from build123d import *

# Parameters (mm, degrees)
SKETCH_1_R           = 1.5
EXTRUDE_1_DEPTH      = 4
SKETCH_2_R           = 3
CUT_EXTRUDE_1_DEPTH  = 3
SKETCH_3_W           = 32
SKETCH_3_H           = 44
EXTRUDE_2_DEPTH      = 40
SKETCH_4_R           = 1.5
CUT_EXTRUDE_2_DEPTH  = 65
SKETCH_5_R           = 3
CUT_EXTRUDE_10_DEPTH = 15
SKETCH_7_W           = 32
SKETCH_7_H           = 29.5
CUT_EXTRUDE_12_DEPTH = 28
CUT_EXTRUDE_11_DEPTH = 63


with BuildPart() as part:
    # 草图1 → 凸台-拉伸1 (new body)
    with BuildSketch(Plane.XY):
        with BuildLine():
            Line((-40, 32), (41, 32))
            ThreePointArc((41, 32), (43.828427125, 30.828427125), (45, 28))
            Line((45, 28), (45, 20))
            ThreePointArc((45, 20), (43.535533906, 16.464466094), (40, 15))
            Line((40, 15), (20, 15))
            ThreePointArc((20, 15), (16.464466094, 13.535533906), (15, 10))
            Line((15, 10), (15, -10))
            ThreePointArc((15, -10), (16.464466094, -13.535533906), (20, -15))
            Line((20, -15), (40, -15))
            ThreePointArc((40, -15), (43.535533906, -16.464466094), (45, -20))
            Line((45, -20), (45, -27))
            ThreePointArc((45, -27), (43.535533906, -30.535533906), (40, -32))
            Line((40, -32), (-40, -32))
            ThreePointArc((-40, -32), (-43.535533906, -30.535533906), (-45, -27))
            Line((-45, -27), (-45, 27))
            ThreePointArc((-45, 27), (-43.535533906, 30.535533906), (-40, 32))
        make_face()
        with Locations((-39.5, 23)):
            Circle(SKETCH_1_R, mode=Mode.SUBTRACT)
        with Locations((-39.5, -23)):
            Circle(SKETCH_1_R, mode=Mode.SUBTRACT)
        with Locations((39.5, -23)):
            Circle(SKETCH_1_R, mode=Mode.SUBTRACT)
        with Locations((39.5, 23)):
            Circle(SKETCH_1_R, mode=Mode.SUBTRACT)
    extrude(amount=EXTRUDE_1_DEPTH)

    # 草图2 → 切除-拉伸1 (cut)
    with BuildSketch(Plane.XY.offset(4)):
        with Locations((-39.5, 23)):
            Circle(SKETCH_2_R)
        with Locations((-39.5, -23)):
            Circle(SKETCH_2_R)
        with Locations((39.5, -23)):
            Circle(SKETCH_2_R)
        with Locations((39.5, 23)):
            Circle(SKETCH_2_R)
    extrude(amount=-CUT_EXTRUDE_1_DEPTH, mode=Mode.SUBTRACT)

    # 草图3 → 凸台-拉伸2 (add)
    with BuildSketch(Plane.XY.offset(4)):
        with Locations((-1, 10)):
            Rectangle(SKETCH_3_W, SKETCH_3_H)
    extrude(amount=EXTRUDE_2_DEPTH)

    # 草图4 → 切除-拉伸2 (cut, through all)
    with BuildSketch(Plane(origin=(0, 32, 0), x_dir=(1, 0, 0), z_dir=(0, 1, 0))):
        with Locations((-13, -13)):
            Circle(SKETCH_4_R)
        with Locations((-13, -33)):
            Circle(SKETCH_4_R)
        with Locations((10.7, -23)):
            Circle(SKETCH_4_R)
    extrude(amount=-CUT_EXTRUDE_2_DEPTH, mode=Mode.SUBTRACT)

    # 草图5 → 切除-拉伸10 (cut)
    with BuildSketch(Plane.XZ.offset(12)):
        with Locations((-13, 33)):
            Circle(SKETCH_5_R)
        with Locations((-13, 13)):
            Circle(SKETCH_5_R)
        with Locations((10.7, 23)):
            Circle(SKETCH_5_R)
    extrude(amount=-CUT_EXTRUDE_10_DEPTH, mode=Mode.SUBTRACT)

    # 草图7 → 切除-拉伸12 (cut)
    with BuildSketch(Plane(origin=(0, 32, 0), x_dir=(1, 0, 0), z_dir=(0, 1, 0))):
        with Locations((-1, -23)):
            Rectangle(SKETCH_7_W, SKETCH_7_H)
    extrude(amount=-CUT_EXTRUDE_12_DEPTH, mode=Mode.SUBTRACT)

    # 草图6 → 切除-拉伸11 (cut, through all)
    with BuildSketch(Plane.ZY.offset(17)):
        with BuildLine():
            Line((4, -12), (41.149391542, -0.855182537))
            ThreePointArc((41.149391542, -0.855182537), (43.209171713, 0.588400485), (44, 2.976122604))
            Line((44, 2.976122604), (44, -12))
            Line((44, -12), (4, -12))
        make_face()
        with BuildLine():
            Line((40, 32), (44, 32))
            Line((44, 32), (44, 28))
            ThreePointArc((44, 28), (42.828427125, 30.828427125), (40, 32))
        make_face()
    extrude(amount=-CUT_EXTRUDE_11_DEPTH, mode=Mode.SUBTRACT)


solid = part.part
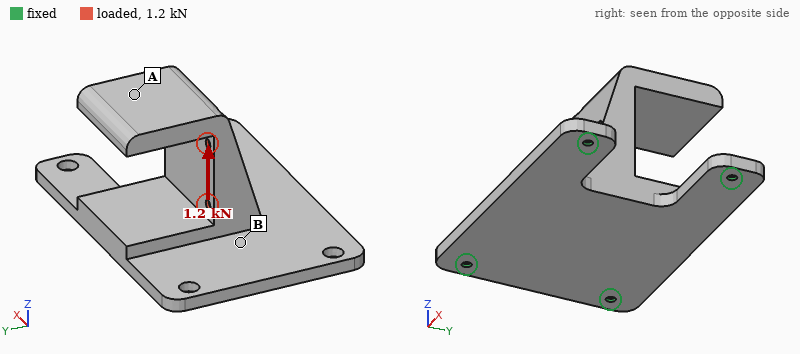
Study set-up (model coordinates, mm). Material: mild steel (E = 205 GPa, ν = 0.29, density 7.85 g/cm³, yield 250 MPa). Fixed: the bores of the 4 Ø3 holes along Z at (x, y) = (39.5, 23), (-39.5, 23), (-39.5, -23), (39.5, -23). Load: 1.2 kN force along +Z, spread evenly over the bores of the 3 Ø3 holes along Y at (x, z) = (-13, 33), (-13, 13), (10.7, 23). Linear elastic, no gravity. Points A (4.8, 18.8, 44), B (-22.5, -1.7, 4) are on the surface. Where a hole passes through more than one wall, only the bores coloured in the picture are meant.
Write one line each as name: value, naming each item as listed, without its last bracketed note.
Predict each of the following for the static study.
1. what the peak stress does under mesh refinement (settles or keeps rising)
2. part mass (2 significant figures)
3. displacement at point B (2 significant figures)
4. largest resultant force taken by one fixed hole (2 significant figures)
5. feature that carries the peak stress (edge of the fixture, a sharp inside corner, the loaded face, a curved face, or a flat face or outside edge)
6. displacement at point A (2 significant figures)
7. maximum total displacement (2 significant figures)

what the peak stress does under mesh refinement: keeps rising
part mass: 320 g
displacement at point B: 39 µm
largest resultant force taken by one fixed hole: 1.1 kN
feature that carries the peak stress: edge of the fixture
displacement at point A: 55 µm
maximum total displacement: 59 µm
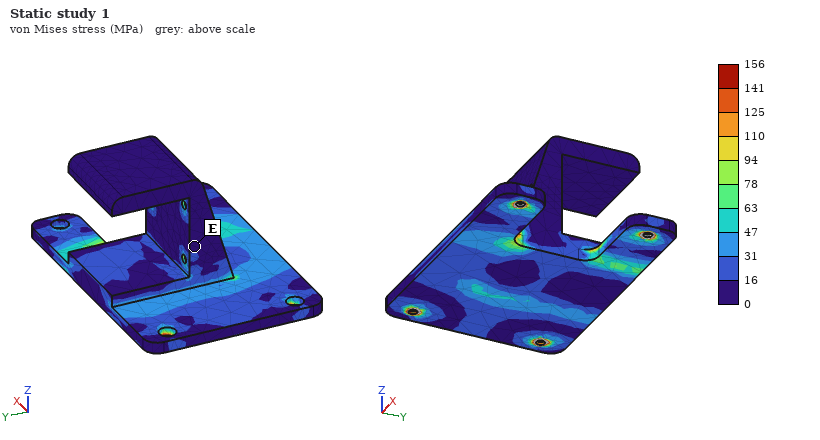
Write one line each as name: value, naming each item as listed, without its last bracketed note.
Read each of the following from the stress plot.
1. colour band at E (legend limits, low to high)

colour band at E: 0 to 16 MPa
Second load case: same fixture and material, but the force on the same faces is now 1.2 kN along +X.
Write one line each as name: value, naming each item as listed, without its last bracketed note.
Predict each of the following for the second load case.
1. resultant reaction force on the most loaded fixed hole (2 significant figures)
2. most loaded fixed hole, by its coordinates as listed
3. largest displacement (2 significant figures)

resultant reaction force on the most loaded fixed hole: 550 N
most loaded fixed hole, by its coordinates as listed: (39.5, 23)
largest displacement: 60 µm
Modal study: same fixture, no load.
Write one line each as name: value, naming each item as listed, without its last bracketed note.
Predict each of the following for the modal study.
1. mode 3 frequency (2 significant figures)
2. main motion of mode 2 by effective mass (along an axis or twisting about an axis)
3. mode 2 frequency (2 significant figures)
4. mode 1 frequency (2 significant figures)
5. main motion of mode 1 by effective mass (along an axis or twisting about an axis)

mode 3 frequency: 2100 Hz
main motion of mode 2 by effective mass: along Z
mode 2 frequency: 1500 Hz
mode 1 frequency: 1400 Hz
main motion of mode 1 by effective mass: along Y
